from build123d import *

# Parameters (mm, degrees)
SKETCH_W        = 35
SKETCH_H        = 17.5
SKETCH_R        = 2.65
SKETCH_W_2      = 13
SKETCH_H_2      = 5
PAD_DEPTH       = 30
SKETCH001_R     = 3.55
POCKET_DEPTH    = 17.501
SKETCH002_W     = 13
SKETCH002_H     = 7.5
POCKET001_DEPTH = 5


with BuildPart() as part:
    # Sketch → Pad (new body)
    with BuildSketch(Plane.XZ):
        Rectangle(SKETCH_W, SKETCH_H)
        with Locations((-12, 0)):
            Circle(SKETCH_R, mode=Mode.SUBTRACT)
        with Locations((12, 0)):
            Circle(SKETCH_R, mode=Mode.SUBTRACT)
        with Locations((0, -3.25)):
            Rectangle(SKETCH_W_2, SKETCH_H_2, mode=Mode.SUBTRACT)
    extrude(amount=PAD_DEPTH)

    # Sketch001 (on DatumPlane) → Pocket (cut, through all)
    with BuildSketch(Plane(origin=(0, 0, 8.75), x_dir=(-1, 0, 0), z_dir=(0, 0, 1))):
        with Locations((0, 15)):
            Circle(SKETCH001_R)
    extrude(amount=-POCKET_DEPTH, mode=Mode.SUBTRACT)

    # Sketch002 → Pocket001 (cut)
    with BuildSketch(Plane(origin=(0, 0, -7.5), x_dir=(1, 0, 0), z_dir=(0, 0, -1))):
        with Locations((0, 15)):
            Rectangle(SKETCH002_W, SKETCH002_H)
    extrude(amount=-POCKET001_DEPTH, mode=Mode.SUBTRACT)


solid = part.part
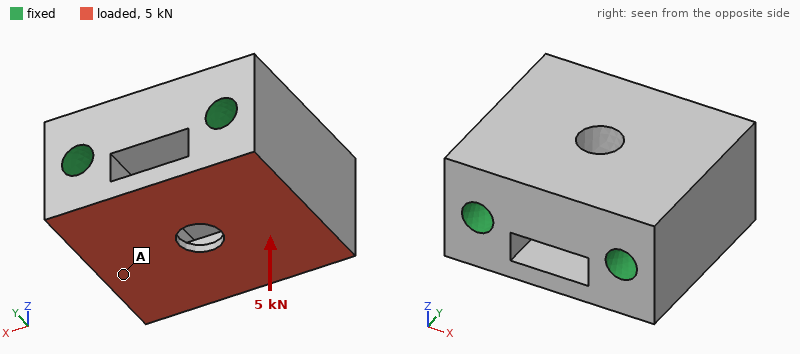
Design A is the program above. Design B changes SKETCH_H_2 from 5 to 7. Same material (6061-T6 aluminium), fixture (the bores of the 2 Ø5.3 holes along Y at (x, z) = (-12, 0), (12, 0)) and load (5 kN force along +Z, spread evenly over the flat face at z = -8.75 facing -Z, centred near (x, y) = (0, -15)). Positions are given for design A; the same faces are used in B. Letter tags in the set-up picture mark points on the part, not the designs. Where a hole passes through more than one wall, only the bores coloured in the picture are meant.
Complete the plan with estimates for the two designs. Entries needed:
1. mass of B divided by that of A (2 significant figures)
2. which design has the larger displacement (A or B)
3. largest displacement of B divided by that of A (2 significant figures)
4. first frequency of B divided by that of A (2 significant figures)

0.96
B
2.0
0.85
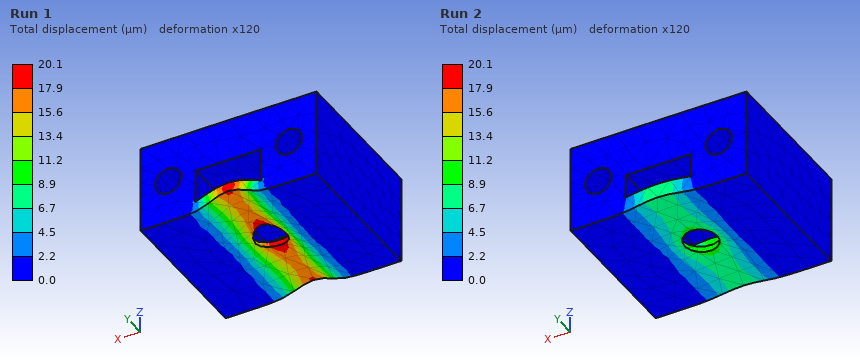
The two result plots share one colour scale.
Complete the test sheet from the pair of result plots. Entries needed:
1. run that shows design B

Run 1
